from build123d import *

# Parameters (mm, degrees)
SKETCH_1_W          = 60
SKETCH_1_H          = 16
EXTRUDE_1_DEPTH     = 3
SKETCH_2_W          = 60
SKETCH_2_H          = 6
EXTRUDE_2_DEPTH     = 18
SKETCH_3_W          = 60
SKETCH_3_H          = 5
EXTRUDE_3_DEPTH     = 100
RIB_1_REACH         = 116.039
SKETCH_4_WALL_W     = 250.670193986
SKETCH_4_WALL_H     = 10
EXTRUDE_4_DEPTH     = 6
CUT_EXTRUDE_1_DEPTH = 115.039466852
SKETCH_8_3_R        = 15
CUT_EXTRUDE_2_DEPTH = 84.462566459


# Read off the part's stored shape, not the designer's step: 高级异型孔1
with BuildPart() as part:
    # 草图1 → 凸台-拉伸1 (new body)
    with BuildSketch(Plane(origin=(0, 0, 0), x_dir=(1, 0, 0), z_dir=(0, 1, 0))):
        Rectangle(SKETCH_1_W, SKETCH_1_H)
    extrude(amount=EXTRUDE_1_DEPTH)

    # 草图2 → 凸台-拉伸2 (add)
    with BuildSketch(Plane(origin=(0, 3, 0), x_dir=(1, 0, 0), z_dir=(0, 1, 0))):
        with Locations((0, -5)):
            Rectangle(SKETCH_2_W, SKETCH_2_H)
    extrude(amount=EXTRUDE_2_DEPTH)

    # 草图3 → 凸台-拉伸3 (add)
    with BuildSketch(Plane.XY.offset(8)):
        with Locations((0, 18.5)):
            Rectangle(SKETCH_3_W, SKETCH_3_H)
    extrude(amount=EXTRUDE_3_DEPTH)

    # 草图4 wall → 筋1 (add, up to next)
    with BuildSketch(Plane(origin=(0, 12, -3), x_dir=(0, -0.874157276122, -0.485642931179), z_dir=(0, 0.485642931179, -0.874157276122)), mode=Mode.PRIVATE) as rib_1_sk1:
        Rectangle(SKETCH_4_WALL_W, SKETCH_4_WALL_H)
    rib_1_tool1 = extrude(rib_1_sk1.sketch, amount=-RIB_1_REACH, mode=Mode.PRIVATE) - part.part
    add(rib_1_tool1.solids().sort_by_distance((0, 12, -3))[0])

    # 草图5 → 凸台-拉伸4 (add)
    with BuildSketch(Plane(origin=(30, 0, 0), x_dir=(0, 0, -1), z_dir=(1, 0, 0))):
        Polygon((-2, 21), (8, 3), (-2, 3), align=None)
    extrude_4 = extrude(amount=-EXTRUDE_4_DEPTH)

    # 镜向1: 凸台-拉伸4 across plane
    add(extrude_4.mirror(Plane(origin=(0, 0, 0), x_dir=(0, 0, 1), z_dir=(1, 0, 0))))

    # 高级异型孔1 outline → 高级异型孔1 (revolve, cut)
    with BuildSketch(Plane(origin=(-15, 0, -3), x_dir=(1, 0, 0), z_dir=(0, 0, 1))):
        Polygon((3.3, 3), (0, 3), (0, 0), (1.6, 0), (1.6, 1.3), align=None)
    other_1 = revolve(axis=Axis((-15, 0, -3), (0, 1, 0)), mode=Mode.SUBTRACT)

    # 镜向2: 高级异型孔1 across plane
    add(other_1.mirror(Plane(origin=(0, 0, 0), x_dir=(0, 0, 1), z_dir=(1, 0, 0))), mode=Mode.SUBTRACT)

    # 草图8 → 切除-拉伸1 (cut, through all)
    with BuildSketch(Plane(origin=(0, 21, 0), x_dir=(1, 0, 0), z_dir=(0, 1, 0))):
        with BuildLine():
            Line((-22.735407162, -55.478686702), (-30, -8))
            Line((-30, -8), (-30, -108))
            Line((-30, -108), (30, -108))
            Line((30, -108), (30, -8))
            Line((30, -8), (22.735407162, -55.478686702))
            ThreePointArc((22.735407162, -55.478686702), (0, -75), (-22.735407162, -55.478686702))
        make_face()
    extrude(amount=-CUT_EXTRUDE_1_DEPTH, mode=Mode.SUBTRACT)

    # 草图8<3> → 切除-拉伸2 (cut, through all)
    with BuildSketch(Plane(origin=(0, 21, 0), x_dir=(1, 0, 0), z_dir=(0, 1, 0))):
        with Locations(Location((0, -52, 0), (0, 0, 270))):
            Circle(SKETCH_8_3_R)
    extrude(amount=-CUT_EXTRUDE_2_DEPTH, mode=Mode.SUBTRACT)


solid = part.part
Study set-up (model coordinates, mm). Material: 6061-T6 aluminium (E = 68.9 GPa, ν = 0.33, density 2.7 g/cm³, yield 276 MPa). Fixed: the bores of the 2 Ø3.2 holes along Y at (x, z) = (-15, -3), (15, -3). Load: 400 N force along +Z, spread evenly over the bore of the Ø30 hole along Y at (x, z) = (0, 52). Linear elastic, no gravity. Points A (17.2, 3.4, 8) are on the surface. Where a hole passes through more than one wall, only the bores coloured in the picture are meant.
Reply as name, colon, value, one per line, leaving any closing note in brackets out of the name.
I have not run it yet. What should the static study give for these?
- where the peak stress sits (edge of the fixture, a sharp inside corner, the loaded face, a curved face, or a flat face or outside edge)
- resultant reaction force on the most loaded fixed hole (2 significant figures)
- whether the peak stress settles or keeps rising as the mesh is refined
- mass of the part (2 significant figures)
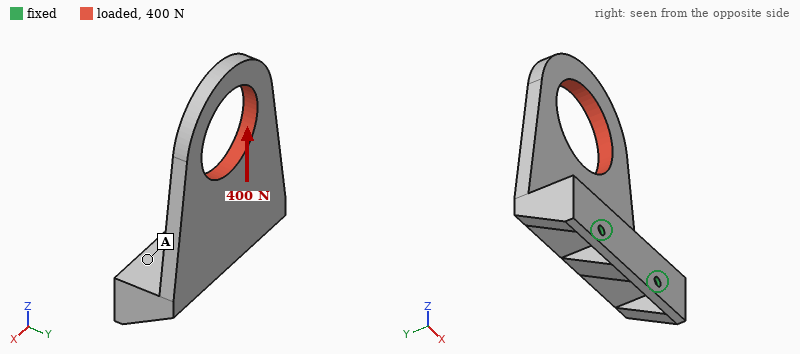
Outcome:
where the peak stress sits: edge of the fixture
resultant reaction force on the most loaded fixed hole: 200 N
whether the peak stress settles or keeps rising as the mesh is refined: keeps rising
mass of the part: 64 g
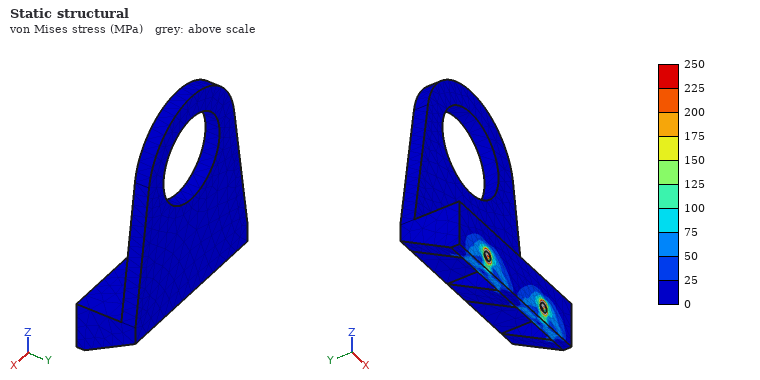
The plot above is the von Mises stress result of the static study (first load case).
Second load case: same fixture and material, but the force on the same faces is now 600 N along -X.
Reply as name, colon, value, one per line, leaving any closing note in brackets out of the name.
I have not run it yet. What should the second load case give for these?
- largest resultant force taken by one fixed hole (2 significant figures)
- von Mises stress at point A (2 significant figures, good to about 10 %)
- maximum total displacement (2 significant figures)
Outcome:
largest resultant force taken by one fixed hole: 1.1 kN
von Mises stress at point A: 29 MPa
maximum total displacement: 0.19 mm
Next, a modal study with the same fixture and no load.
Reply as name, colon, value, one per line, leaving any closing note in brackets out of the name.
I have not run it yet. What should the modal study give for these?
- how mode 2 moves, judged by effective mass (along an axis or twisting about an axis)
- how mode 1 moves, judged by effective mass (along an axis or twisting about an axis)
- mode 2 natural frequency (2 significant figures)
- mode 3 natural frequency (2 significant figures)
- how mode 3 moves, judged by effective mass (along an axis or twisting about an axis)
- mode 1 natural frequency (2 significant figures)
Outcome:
how mode 2 moves, judged by effective mass: along X
how mode 1 moves, judged by effective mass: along Y
mode 2 natural frequency: 2200 Hz
mode 3 natural frequency: 2300 Hz
how mode 3 moves, judged by effective mass: along Z
mode 1 natural frequency: 490 Hz
